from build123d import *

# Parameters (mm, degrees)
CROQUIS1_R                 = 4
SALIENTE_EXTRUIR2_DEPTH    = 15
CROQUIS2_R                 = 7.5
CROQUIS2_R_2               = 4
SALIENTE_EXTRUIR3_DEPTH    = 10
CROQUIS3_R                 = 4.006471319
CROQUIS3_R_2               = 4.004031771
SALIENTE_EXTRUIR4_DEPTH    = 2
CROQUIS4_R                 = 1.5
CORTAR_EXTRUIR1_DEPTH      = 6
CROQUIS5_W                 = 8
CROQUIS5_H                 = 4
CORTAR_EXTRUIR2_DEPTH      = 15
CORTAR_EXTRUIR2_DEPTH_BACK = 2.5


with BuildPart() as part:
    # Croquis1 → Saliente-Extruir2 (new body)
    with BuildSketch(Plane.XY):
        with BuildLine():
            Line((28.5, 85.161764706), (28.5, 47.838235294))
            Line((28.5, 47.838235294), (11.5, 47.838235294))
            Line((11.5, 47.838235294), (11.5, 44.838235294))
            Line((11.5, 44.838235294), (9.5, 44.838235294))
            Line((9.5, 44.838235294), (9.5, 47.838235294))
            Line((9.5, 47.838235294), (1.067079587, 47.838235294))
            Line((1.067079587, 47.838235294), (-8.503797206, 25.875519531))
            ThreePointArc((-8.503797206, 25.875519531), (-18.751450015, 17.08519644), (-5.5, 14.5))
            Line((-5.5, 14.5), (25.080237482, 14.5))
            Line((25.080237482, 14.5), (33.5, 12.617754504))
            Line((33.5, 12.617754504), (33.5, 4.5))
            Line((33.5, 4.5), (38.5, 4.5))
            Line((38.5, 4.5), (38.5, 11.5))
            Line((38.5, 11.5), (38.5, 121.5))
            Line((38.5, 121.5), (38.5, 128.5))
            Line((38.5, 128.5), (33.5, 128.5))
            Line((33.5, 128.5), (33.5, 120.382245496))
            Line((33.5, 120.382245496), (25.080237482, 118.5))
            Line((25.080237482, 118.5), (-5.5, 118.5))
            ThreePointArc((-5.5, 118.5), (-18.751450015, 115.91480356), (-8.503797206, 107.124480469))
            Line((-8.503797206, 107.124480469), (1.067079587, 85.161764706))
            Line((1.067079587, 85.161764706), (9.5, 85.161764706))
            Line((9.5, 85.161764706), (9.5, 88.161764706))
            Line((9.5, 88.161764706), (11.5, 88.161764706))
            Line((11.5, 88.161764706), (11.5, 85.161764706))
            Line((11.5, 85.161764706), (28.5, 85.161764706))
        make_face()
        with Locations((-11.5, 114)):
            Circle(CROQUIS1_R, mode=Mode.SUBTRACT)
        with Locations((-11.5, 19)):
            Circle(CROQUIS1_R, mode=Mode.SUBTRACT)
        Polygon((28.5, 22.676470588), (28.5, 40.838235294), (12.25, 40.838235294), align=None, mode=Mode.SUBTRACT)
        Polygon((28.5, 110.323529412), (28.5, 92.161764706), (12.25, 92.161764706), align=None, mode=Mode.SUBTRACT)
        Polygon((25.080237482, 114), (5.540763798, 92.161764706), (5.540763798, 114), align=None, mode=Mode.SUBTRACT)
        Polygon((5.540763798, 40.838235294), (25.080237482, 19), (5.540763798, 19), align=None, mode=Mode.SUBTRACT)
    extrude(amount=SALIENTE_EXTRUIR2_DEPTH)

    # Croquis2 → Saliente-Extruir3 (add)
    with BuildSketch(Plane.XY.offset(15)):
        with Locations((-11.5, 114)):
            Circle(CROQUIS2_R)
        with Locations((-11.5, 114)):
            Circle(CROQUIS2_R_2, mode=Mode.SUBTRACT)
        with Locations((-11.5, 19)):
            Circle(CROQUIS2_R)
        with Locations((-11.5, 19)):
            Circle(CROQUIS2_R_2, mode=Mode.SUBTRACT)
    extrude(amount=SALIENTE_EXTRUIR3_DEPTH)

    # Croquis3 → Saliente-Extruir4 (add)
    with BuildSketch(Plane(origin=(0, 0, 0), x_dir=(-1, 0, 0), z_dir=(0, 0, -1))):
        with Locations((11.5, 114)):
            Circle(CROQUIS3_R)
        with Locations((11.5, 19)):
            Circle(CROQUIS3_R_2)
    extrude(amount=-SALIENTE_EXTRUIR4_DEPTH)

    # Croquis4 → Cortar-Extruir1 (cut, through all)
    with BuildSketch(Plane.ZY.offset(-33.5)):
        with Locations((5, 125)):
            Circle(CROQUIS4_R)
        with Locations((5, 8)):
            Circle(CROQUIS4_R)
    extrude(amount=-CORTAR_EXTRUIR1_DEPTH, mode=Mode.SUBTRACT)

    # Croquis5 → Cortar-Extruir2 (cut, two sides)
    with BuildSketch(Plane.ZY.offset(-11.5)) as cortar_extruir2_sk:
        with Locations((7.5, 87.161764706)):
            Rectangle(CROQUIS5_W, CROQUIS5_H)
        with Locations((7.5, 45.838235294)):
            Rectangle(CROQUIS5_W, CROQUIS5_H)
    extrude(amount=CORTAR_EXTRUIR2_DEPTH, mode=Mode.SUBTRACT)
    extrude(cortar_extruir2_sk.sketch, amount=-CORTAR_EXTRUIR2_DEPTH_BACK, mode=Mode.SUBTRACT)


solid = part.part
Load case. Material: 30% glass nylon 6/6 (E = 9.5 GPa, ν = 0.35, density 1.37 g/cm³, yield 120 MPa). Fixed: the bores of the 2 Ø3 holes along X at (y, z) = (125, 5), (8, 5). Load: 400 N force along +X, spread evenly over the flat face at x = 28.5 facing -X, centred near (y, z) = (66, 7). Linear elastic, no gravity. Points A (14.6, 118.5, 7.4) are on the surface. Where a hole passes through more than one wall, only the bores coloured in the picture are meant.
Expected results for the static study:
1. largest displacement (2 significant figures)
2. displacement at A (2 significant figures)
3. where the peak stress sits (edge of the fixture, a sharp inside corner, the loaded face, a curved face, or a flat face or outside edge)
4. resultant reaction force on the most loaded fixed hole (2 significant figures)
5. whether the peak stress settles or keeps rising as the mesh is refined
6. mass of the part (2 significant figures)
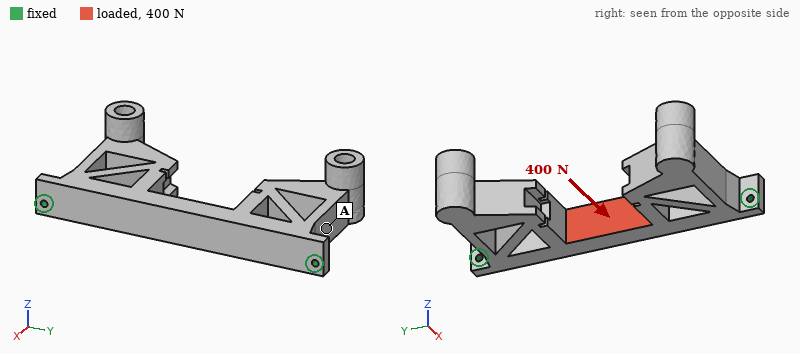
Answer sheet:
0.61 mm
0.23 mm
edge of the fixture
500 N
keeps rising
61 g
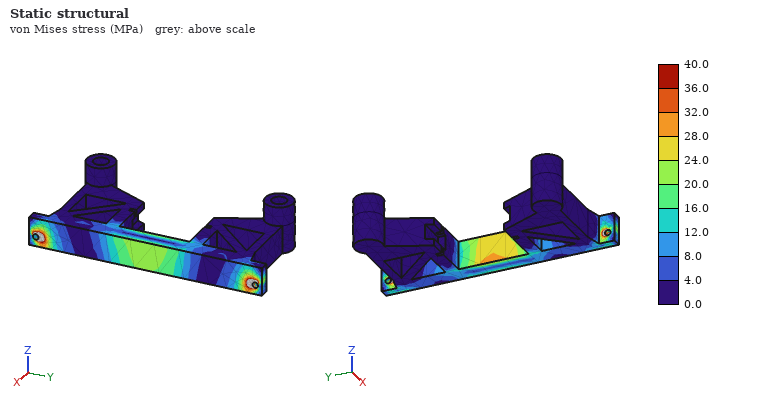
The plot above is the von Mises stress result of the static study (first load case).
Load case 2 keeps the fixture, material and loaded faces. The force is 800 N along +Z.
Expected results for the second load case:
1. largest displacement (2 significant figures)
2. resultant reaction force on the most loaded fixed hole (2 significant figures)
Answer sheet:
0.93 mm
600 N
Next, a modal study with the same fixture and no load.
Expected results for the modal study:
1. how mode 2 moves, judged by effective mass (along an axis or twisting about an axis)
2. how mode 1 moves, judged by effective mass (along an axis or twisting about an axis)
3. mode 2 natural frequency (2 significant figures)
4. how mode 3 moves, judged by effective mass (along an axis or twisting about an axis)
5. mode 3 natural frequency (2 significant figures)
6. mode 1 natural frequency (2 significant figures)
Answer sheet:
along X
along Z
710 Hz
twisting about X
830 Hz
500 Hz
